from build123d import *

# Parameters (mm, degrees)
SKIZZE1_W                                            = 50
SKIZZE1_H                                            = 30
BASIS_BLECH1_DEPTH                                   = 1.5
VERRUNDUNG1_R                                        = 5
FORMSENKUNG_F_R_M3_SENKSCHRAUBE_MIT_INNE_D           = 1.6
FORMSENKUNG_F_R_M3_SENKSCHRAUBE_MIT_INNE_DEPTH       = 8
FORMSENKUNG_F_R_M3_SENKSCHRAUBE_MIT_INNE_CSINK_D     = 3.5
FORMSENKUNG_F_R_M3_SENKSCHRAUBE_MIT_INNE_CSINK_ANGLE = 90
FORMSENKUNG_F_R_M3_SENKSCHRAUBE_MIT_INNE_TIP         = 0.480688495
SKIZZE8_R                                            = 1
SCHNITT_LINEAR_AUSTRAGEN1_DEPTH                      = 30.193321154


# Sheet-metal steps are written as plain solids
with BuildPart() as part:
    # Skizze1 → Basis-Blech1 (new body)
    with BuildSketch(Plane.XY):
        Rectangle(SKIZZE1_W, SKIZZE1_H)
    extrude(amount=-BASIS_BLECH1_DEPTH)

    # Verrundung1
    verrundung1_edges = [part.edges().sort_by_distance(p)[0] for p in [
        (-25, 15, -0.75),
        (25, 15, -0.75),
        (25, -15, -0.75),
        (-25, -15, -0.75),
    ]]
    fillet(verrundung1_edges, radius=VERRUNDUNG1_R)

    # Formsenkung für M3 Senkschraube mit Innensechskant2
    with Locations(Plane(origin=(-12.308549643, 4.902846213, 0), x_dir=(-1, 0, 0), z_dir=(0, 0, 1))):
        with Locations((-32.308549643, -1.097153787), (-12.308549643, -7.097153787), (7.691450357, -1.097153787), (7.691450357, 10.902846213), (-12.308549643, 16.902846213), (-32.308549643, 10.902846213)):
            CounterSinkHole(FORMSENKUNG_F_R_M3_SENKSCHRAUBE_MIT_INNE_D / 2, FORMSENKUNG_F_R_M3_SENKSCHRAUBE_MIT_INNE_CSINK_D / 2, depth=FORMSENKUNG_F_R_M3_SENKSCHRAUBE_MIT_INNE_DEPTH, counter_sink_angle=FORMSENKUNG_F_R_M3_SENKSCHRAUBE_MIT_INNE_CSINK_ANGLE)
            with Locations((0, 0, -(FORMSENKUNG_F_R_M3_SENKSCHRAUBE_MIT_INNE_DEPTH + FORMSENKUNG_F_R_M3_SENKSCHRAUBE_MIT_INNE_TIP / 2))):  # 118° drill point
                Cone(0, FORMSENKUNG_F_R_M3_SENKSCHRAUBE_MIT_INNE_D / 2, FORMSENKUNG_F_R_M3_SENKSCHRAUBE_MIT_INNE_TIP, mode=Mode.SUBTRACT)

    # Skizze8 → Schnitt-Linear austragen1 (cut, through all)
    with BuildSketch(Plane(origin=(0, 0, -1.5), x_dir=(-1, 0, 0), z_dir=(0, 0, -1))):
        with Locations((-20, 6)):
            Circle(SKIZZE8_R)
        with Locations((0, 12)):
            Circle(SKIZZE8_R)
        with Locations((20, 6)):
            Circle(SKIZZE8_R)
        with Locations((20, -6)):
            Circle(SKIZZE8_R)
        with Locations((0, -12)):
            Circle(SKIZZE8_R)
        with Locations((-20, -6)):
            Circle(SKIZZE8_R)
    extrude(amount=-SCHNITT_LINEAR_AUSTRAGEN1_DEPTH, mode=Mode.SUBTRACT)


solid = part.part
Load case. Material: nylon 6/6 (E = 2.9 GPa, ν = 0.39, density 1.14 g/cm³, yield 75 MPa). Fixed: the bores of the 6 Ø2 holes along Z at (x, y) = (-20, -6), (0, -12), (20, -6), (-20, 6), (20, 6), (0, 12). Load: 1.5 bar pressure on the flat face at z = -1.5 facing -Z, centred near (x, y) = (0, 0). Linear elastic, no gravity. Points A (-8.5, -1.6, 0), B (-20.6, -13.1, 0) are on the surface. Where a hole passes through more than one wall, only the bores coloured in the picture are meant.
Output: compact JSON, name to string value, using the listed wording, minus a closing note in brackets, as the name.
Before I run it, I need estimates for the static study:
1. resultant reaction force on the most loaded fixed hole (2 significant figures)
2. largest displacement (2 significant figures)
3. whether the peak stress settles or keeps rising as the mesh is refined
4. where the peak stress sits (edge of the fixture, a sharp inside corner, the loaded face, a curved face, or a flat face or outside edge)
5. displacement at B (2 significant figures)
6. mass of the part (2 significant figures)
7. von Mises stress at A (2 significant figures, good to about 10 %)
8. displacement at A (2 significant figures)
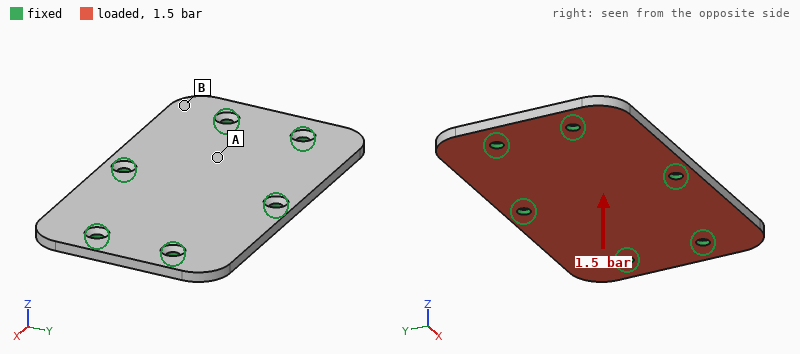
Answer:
{"resultant reaction force on the most loaded fixed hole": "50 N", "largest displacement": "0.22 mm", "whether the peak stress settles or keeps rising as the mesh is refined": "keeps rising", "where the peak stress sits": "edge of the fixture", "displacement at B": "0.11 mm", "mass of the part": "2.5 g", "von Mises stress at A": "7.8 MPa", "displacement at A": "0.20 mm"}
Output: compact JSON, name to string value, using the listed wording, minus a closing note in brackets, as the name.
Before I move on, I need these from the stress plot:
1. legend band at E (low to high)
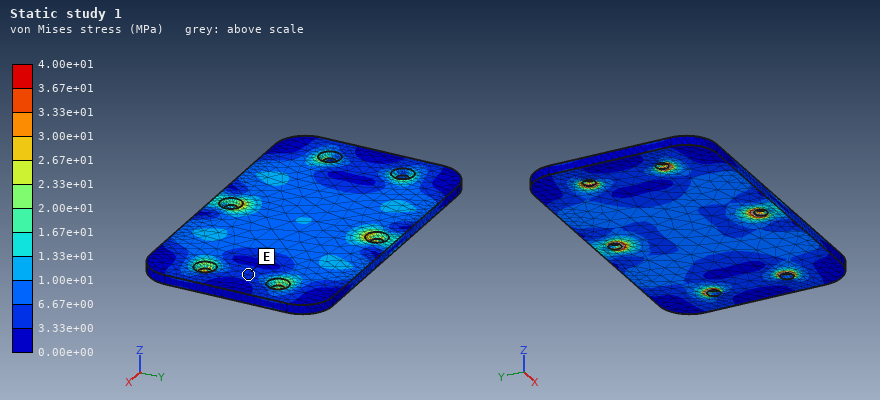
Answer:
{"legend band at E": "3.33e+00 to 6.67e+00 MPa"}
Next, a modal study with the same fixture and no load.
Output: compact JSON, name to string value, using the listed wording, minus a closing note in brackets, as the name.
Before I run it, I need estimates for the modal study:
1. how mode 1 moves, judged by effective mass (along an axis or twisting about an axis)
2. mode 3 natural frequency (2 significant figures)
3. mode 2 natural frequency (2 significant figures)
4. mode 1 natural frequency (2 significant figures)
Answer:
{"how mode 1 moves, judged by effective mass": "along Z", "mode 3 natural frequency": "4000 Hz", "mode 2 natural frequency": "3900 Hz", "mode 1 natural frequency": "3600 Hz"}
